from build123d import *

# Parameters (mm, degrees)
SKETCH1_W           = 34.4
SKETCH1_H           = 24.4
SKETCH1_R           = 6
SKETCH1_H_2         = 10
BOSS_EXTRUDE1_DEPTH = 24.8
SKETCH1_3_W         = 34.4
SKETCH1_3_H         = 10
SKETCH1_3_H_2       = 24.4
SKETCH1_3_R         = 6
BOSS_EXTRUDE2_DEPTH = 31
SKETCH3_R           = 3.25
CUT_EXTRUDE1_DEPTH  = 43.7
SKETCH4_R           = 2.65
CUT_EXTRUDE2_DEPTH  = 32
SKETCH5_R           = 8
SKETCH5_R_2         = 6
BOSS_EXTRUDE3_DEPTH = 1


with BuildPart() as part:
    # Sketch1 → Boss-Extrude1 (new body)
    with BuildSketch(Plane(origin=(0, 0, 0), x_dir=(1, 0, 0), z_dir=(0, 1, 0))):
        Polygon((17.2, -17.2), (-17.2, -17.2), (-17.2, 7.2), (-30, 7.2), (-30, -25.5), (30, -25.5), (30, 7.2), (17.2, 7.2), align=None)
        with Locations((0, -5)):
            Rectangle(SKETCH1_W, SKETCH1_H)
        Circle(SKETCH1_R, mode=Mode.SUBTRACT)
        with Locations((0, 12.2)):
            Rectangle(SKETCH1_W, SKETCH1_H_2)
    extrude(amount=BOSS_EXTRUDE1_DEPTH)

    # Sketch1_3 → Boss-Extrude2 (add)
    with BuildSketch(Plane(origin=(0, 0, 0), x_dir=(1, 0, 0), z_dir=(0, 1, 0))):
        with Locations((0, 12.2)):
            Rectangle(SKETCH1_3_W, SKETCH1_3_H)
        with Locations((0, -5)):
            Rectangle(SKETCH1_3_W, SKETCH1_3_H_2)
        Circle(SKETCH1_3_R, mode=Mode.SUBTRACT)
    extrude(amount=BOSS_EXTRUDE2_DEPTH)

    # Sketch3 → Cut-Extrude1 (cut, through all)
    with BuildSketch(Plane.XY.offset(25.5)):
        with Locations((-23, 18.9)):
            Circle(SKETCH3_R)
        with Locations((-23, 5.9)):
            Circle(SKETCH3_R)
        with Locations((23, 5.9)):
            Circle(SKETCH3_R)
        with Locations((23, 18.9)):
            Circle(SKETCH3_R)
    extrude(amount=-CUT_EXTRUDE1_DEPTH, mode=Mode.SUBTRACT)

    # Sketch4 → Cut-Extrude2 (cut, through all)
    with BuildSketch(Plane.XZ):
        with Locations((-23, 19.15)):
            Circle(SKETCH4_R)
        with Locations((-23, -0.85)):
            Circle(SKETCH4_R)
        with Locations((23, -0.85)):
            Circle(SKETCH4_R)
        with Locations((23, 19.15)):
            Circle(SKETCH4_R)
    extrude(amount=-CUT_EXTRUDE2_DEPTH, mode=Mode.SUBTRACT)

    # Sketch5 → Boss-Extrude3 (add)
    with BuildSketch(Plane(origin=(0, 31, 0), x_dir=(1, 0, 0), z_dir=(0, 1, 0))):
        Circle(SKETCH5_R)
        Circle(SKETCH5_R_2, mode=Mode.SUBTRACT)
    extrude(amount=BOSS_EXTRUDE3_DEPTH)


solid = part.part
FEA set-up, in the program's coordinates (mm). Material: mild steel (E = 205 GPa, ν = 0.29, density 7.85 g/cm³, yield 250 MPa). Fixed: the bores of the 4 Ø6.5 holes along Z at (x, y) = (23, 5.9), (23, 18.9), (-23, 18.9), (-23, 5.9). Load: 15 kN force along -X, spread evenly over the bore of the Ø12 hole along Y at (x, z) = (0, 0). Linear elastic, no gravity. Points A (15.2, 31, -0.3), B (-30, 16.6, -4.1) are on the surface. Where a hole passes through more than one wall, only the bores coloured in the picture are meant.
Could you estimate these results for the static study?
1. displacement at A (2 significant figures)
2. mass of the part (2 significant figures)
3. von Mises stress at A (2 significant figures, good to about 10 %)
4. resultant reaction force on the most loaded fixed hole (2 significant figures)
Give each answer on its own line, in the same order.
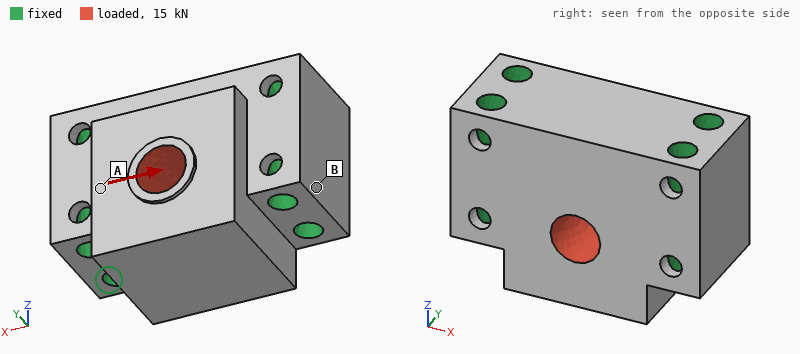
1.3 µm
440 g
8.1 MPa
4.3 kN
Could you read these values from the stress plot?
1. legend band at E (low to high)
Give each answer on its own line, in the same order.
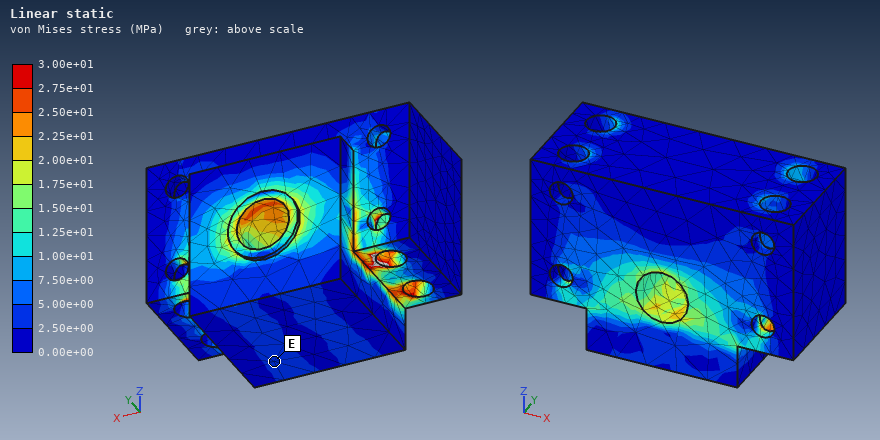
2.50e+00 to 5.00e+00 MPa
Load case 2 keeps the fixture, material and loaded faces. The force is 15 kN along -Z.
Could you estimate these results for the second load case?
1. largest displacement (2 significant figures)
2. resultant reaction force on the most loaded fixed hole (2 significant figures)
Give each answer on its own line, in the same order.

3.8 µm
4.6 kN
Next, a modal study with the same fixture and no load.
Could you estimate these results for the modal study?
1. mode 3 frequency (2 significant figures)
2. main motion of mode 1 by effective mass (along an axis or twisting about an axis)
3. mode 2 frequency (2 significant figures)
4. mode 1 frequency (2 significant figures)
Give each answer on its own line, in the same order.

32 kHz
along Y
30 kHz
20 kHz
